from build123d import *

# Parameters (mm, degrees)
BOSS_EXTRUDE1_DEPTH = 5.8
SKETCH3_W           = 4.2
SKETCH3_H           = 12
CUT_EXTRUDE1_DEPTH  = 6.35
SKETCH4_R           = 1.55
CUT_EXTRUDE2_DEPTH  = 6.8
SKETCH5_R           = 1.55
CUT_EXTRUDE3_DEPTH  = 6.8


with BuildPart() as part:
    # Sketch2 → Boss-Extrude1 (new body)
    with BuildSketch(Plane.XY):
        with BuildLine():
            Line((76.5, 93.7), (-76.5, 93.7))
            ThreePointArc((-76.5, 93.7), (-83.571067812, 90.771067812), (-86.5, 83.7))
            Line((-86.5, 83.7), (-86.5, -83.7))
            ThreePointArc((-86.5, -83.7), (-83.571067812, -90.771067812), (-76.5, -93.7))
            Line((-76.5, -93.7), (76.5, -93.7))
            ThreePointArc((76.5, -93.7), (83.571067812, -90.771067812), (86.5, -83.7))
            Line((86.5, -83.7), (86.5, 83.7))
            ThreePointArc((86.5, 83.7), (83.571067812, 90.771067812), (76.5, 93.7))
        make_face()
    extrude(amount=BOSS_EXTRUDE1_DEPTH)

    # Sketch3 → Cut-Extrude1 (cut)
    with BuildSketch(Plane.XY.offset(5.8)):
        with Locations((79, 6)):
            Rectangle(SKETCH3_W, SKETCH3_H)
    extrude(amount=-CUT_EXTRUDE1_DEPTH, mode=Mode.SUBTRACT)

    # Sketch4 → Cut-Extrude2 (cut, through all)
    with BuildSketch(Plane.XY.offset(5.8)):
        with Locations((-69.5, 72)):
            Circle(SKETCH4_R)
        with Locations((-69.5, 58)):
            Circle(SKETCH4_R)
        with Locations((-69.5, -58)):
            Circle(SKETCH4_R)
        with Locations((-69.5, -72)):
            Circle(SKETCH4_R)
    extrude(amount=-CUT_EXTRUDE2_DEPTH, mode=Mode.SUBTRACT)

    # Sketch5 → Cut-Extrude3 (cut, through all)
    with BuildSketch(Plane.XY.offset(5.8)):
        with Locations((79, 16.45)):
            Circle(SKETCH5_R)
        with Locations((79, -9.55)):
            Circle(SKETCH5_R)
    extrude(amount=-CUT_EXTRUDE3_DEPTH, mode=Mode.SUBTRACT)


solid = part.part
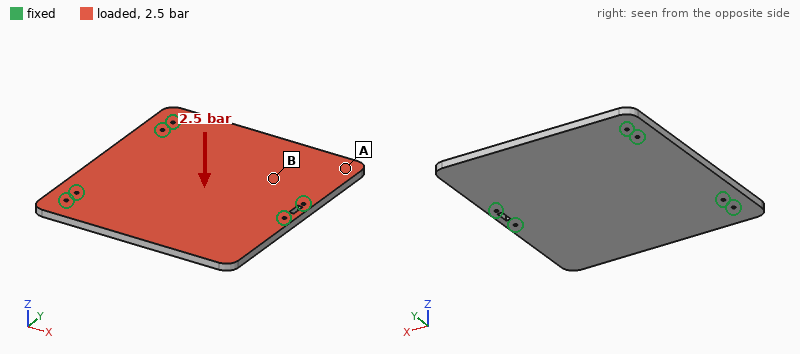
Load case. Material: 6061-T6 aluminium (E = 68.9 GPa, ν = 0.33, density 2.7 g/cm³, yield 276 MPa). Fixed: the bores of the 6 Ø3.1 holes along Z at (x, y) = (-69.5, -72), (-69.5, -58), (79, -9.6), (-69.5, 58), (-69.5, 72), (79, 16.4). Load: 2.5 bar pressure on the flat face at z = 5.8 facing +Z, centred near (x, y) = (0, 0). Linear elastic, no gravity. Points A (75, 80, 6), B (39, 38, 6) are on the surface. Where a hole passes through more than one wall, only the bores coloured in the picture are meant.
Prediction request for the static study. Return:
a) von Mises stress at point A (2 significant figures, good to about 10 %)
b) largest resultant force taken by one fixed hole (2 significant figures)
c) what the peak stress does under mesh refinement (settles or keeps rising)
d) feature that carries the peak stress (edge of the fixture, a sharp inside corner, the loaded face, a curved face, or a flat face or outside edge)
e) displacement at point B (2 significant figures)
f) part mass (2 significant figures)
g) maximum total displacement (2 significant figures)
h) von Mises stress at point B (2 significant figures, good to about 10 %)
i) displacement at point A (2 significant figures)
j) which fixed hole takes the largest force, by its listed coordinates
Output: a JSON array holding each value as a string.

["20 MPa", "1.9 kN", "keeps rising", "edge of the fixture", "0.50 mm", "500 g", "1.3 mm", "59 MPa", "0.82 mm", "(79, -9.6)"]
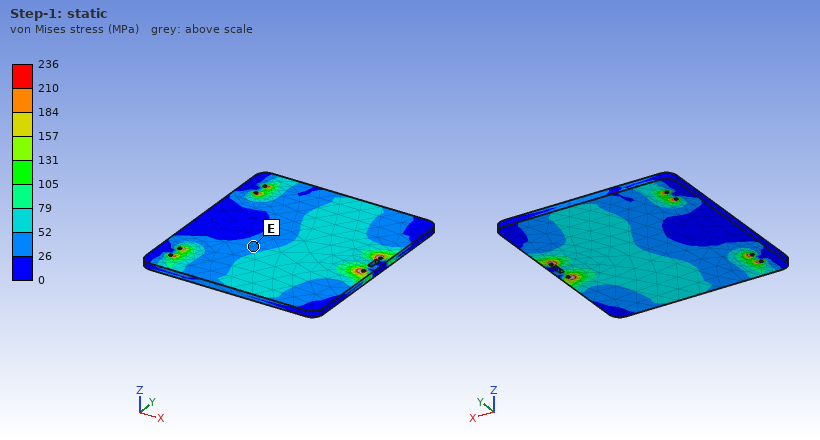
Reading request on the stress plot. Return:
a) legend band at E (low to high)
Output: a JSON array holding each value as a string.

["26 to 52 MPa"]
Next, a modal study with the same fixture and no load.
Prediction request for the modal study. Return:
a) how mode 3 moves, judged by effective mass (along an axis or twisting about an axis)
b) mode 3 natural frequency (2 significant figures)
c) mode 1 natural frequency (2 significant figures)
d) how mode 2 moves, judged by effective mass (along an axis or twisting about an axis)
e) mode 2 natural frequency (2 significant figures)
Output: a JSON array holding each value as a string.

["along Z", "1200 Hz", "690 Hz", "along Z", "770 Hz"]
